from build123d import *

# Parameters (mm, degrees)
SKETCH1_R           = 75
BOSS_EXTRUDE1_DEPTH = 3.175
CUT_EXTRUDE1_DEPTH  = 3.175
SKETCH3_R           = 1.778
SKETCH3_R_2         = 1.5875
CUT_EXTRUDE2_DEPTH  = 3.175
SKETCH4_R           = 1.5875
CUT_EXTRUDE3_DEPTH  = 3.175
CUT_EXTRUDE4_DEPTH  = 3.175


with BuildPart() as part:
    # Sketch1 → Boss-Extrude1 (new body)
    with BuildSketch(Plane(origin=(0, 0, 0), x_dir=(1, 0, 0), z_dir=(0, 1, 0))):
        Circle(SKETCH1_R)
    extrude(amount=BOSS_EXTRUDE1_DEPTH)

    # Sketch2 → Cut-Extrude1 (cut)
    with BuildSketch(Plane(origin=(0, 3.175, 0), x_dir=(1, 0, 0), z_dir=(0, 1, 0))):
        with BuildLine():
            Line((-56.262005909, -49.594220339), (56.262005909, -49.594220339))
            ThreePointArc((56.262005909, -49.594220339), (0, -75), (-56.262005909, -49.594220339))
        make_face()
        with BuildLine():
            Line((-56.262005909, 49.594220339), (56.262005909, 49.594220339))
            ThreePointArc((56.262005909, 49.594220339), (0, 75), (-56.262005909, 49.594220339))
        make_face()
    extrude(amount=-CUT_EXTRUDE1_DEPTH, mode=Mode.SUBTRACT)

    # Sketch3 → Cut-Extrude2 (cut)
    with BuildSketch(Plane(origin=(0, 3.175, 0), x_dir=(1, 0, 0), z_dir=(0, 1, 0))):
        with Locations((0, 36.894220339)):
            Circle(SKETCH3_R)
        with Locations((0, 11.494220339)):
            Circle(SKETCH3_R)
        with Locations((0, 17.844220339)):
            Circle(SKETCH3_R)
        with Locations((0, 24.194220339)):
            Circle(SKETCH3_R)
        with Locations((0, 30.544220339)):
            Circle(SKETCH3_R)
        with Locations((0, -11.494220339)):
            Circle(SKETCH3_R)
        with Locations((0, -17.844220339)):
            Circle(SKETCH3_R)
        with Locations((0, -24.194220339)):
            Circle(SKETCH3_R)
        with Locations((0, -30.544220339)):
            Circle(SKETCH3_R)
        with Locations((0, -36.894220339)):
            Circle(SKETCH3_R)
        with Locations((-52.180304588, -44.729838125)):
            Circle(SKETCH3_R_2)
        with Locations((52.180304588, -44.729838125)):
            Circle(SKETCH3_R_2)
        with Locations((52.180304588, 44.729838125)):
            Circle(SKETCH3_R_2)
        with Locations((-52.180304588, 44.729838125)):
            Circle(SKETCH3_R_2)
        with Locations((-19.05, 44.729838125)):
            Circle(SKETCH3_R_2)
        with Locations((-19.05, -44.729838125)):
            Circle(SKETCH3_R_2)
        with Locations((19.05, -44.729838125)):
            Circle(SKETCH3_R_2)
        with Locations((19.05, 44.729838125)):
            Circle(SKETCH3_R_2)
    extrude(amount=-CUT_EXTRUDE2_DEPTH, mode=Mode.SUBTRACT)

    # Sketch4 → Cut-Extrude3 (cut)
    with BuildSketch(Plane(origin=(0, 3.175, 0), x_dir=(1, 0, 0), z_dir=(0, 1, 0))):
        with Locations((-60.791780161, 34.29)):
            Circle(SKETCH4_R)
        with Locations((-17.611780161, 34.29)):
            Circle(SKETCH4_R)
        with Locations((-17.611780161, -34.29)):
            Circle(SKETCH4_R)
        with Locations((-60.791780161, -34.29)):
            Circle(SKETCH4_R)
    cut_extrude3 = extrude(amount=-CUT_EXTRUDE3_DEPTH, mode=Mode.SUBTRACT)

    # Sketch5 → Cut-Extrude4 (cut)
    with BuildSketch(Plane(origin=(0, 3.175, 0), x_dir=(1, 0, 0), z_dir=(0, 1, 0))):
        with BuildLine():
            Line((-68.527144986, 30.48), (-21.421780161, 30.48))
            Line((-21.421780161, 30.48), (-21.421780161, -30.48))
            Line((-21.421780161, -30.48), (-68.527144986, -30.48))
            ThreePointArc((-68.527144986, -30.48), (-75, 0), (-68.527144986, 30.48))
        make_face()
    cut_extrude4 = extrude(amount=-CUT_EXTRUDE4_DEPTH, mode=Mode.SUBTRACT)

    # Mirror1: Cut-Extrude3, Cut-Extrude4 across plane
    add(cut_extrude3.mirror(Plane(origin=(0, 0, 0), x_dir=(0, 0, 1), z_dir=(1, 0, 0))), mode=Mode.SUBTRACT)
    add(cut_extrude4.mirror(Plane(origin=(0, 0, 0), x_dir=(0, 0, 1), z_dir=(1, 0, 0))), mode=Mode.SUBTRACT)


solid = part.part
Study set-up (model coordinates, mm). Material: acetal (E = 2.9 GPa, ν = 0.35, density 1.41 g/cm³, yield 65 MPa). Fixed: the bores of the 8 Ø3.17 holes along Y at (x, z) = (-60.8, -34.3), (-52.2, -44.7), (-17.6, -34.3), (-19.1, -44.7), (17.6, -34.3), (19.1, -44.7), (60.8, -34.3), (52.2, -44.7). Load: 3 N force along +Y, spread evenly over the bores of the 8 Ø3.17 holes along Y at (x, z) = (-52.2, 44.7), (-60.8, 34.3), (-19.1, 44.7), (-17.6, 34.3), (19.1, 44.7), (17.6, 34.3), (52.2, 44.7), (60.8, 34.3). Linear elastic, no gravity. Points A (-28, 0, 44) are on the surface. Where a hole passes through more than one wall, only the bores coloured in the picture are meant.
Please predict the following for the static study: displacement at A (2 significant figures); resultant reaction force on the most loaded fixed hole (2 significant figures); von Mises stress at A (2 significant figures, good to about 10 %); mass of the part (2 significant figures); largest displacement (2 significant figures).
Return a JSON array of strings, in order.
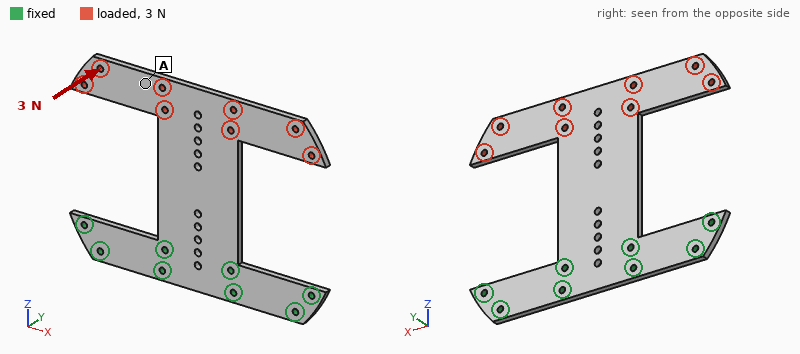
["1.5 mm", "5.9 N", "0.62 MPa", "32 g", "1.7 mm"]
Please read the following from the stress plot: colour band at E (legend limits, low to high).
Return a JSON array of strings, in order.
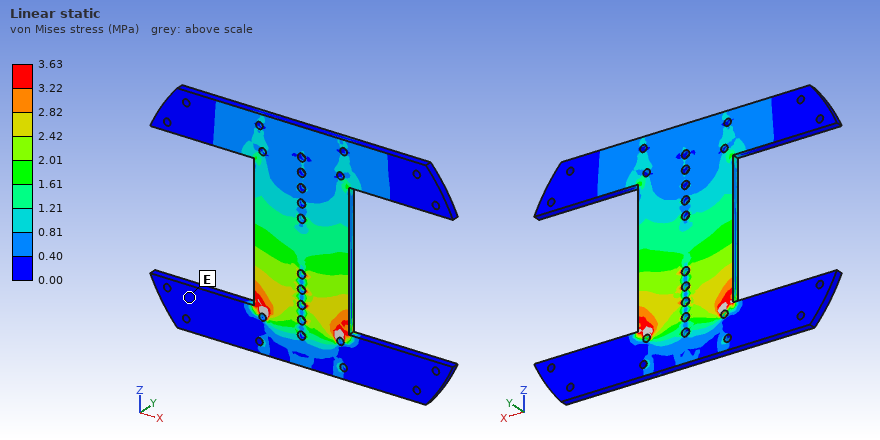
["0.00 to 0.40 MPa"]
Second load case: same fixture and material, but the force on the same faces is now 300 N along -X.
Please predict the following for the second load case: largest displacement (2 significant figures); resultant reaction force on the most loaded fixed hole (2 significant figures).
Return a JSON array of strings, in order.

["1.3 mm", "520 N"]
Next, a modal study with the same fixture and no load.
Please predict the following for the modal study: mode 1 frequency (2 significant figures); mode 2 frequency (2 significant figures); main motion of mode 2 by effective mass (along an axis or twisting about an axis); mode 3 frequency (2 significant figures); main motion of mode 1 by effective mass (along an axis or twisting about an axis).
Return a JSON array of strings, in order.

["67 Hz", "110 Hz", "twisting about Z", "310 Hz", "along Y"]
